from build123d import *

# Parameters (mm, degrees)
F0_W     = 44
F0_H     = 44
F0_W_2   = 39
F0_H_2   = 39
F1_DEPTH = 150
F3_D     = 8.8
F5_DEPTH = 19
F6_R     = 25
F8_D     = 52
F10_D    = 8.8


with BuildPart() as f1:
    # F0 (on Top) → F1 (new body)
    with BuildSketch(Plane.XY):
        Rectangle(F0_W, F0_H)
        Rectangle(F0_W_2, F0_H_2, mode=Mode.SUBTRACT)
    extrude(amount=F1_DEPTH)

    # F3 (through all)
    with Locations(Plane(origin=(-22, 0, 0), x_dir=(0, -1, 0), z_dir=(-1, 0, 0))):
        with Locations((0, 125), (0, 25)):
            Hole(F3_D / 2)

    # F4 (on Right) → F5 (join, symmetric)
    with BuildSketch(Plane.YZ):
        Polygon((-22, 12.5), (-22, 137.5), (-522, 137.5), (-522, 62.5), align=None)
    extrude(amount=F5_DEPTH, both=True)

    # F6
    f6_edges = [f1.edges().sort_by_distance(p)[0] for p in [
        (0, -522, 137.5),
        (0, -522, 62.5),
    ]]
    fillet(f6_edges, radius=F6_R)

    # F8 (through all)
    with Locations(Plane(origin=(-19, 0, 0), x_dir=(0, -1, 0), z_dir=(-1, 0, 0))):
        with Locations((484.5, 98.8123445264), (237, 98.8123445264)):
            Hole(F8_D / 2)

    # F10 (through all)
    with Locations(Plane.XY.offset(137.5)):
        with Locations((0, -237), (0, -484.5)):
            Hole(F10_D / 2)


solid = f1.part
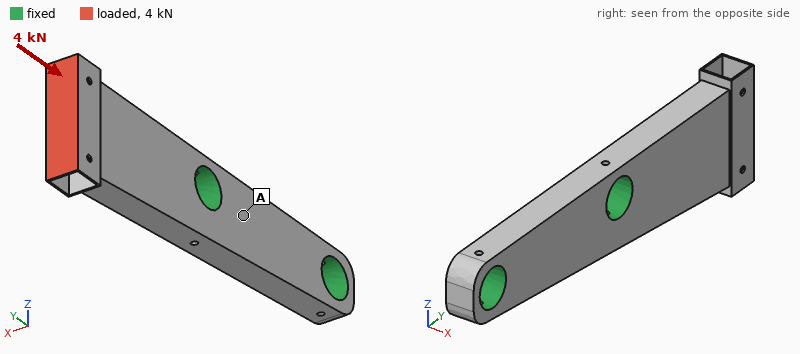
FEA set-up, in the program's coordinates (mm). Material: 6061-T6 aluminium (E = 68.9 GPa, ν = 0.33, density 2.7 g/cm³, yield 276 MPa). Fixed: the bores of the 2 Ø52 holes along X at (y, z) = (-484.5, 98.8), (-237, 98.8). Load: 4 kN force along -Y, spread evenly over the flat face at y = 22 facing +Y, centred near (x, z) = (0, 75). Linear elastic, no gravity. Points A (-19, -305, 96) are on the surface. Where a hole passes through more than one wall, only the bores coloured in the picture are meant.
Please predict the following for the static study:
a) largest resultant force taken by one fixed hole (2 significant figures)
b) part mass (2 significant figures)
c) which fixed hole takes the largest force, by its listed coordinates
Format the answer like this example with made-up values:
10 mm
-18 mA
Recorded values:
3.8 kN
4.8 kg
(-237, 98.8)
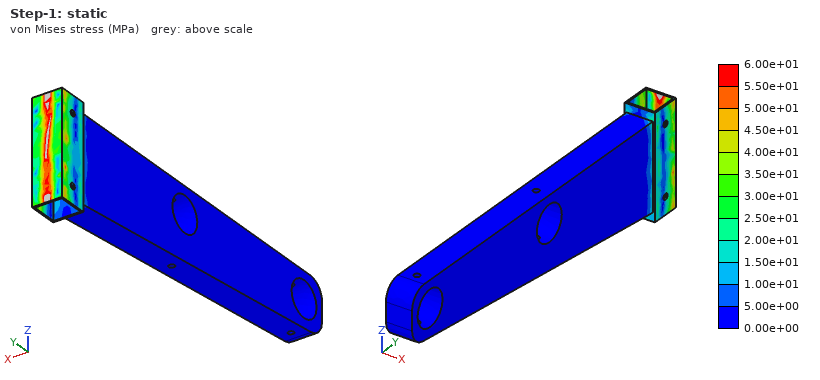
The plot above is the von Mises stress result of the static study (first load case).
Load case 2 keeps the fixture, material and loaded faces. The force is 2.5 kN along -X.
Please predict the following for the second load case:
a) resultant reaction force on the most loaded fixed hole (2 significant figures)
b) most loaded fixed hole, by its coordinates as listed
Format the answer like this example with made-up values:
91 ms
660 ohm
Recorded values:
2.5 kN
(-237, 98.8)
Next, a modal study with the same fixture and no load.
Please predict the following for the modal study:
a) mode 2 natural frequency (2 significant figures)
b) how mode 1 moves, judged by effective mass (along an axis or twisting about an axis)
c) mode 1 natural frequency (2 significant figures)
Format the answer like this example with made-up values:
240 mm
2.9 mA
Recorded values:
1300 Hz
along X
610 Hz
